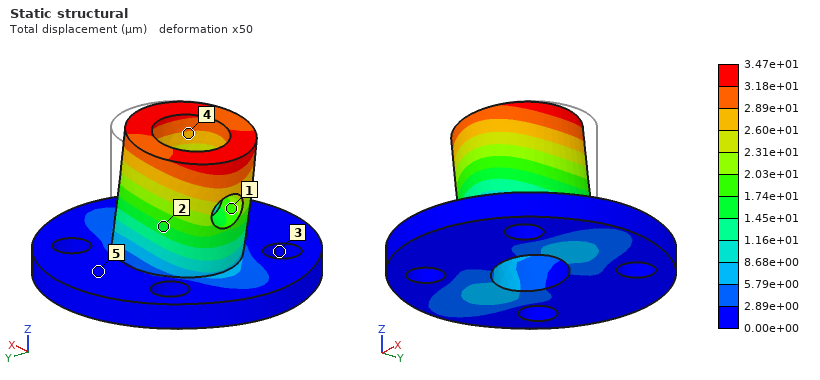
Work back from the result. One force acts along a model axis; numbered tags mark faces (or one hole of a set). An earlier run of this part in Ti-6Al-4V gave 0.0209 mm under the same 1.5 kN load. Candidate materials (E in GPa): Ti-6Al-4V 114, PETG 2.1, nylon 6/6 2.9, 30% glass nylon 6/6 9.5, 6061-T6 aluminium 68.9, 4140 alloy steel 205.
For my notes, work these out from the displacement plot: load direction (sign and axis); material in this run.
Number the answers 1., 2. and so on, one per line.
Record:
1. -X
2. 6061-T6 aluminium
